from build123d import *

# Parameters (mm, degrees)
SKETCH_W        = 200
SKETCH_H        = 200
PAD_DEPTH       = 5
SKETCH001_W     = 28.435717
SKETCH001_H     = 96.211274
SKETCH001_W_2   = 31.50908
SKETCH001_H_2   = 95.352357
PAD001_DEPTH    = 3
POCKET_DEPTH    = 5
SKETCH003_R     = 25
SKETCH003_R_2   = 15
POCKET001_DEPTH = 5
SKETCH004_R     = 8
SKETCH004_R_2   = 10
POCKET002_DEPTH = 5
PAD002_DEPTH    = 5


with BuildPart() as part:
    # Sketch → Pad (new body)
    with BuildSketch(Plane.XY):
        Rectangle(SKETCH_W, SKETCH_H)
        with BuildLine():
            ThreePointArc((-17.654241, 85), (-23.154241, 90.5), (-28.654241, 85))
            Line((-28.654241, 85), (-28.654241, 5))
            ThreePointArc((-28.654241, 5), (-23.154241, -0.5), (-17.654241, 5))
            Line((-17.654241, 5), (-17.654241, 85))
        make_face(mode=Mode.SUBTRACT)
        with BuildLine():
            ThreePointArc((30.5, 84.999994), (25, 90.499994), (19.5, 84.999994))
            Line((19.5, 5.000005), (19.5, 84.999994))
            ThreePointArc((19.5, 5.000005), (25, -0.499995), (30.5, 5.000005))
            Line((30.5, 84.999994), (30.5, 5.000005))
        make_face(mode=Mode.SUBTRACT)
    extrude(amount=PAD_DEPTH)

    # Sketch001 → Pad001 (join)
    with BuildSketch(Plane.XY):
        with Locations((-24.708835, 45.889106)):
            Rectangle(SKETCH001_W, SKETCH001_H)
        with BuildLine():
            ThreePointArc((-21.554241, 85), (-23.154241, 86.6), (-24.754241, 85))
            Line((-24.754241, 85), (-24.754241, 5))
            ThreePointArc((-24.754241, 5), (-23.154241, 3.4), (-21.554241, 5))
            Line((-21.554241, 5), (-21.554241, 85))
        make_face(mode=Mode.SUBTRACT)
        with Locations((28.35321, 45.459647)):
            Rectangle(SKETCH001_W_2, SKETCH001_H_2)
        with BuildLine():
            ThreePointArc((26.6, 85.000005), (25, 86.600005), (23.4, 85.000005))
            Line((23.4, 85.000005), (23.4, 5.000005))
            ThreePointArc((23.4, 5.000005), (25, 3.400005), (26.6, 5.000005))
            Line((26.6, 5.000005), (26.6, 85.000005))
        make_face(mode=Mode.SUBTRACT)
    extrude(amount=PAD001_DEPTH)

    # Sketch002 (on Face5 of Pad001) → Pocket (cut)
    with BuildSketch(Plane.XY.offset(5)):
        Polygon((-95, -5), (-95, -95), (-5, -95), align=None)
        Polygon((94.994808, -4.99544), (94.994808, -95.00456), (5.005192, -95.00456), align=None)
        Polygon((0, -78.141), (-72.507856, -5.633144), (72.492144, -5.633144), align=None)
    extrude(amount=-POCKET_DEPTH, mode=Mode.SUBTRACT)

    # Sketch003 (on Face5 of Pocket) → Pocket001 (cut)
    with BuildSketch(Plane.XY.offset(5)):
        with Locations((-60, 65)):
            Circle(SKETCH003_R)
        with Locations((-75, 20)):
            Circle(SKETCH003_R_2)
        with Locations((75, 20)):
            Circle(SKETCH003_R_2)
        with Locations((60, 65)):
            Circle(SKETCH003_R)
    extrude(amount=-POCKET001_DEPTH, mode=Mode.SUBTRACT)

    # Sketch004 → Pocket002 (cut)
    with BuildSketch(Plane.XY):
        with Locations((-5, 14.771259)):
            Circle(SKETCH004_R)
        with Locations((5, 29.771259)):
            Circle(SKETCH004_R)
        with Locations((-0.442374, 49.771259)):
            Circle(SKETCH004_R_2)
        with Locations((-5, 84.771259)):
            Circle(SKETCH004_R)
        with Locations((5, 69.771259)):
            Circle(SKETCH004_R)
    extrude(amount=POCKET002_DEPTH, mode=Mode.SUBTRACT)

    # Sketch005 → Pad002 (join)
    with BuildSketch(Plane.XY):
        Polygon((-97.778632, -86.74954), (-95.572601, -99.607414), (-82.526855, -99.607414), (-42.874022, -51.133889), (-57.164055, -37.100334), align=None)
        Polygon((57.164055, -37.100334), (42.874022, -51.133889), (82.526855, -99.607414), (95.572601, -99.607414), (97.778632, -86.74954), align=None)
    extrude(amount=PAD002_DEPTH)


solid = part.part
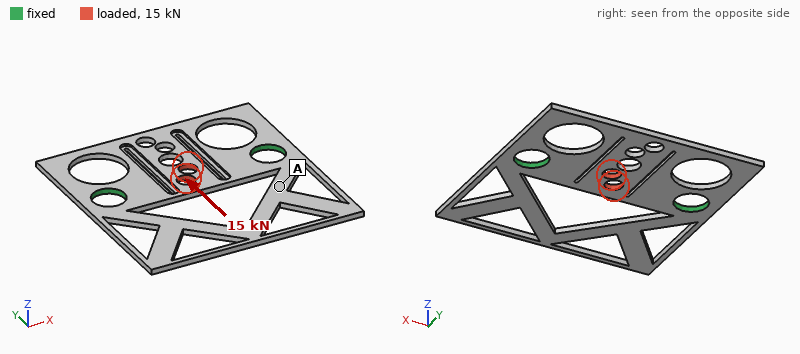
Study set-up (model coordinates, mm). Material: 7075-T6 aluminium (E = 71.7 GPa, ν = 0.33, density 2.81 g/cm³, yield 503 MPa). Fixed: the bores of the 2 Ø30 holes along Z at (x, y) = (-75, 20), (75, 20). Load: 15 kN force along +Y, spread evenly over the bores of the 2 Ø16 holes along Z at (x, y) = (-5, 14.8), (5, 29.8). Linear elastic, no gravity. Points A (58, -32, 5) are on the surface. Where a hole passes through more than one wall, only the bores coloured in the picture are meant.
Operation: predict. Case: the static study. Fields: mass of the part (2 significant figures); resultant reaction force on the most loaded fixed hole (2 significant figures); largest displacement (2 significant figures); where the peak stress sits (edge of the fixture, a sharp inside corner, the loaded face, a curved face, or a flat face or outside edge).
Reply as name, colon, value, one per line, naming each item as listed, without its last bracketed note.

mass of the part: 300 g
resultant reaction force on the most loaded fixed hole: 7.6 kN
largest displacement: 0.29 mm
where the peak stress sits: a curved face
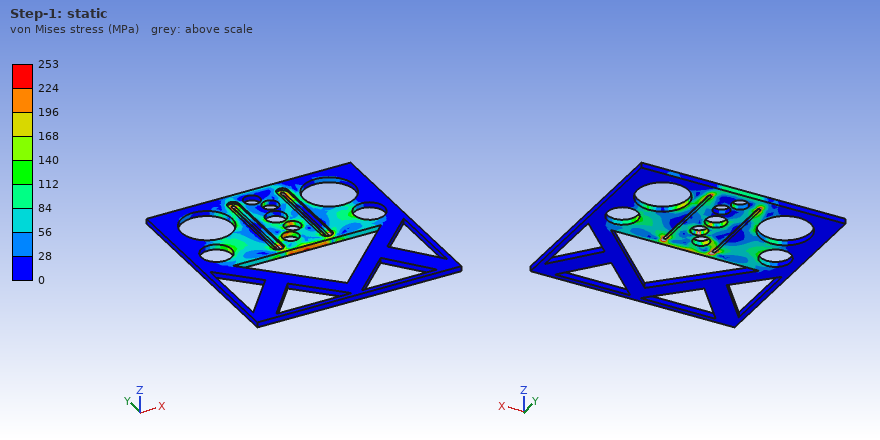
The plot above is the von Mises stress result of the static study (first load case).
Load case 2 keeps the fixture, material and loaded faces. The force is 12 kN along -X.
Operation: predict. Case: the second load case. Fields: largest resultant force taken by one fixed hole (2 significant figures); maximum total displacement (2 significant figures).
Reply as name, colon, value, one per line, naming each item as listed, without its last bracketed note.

largest resultant force taken by one fixed hole: 6.2 kN
maximum total displacement: 0.23 mm
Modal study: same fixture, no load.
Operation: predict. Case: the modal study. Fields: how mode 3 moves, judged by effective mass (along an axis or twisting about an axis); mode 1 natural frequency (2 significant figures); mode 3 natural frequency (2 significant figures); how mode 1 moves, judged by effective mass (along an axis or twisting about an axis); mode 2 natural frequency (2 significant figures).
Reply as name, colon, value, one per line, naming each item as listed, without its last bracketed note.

how mode 3 moves, judged by effective mass: along Z
mode 1 natural frequency: 230 Hz
mode 3 natural frequency: 530 Hz
how mode 1 moves, judged by effective mass: along Z
mode 2 natural frequency: 400 Hz
